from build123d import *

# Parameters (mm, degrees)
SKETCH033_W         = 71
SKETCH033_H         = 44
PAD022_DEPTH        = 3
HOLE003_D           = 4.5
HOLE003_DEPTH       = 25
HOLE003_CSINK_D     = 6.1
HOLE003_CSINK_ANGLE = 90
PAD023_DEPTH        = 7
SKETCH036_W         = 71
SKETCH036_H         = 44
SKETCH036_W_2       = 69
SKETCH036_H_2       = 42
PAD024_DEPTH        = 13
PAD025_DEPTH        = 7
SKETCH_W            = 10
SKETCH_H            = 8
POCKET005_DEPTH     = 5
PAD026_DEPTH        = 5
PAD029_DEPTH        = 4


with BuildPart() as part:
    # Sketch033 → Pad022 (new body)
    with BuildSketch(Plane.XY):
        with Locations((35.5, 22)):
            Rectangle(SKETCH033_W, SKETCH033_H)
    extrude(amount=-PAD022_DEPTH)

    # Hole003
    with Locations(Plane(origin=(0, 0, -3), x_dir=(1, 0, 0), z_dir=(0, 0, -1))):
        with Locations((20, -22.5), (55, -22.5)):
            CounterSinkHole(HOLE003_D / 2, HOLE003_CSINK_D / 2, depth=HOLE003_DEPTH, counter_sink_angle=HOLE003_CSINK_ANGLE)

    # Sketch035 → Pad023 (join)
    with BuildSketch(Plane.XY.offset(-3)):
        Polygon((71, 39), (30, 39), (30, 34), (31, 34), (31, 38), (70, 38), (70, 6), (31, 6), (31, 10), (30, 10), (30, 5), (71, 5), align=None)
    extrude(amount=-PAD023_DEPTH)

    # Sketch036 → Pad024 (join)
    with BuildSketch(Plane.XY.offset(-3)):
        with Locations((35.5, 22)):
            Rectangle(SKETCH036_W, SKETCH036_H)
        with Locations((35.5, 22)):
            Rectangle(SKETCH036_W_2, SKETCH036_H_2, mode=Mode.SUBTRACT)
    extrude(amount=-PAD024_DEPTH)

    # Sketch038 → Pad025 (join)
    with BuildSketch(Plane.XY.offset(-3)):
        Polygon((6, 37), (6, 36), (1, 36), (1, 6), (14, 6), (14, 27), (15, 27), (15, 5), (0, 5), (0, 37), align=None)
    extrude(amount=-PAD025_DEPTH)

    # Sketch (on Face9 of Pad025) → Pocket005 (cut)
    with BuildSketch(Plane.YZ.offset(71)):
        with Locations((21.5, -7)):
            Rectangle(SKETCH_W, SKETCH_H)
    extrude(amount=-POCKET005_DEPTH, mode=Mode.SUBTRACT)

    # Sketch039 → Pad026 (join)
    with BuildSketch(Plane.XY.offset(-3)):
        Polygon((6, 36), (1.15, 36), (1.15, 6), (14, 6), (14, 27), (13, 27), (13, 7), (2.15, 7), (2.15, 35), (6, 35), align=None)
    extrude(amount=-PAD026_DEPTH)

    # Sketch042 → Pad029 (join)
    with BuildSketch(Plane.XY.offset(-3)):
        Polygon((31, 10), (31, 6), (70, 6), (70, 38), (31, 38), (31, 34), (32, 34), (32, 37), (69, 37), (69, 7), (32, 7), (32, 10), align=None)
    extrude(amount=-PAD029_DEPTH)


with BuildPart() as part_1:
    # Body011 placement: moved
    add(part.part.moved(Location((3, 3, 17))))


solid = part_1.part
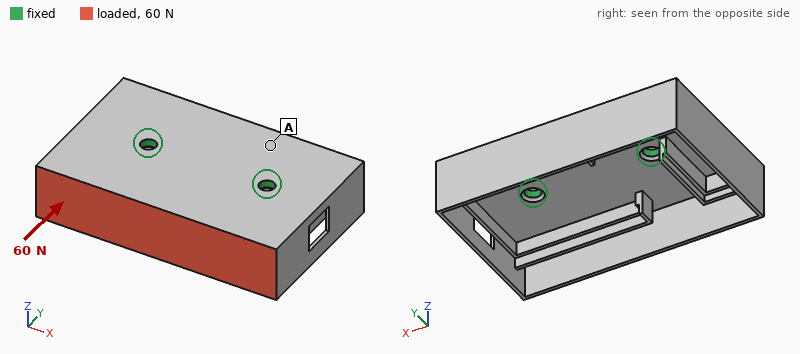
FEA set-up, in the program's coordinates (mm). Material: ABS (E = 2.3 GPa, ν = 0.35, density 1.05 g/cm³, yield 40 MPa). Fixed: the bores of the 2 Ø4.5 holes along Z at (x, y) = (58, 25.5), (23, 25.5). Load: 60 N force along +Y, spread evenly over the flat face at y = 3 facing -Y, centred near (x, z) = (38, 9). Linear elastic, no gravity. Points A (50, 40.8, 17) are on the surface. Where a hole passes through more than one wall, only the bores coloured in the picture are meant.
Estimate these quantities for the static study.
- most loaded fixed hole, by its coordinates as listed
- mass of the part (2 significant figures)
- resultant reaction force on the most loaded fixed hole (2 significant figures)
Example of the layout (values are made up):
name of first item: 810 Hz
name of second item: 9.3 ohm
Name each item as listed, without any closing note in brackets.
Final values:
most loaded fixed hole, by its coordinates as listed: (23, 25.5)
mass of the part: 14 g
resultant reaction force on the most loaded fixed hole: 34 N
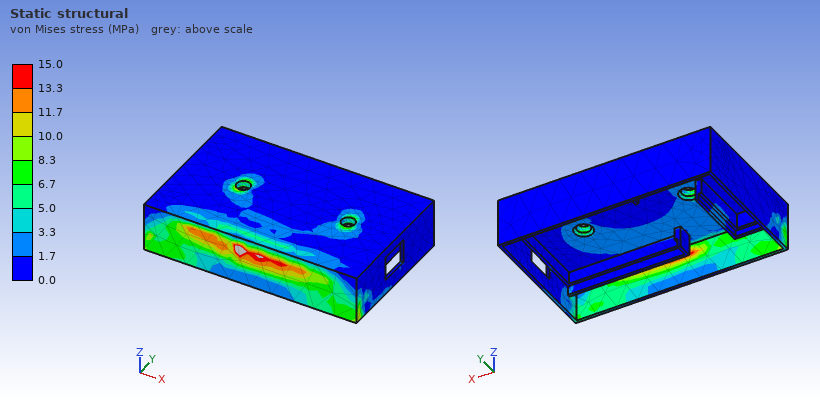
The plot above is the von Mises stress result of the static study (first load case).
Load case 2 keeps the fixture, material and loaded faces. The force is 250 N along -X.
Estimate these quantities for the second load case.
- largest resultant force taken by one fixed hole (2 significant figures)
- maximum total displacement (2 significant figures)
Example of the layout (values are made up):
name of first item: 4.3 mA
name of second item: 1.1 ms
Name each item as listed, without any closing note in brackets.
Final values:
largest resultant force taken by one fixed hole: 200 N
maximum total displacement: 0.89 mm
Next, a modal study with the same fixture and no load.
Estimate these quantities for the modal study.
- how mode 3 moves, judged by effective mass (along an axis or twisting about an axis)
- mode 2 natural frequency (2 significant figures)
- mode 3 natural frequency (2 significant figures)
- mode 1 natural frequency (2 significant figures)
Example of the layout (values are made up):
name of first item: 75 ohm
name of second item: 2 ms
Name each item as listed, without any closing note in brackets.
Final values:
how mode 3 moves, judged by effective mass: along Z
mode 2 natural frequency: 870 Hz
mode 3 natural frequency: 1200 Hz
mode 1 natural frequency: 740 Hz
